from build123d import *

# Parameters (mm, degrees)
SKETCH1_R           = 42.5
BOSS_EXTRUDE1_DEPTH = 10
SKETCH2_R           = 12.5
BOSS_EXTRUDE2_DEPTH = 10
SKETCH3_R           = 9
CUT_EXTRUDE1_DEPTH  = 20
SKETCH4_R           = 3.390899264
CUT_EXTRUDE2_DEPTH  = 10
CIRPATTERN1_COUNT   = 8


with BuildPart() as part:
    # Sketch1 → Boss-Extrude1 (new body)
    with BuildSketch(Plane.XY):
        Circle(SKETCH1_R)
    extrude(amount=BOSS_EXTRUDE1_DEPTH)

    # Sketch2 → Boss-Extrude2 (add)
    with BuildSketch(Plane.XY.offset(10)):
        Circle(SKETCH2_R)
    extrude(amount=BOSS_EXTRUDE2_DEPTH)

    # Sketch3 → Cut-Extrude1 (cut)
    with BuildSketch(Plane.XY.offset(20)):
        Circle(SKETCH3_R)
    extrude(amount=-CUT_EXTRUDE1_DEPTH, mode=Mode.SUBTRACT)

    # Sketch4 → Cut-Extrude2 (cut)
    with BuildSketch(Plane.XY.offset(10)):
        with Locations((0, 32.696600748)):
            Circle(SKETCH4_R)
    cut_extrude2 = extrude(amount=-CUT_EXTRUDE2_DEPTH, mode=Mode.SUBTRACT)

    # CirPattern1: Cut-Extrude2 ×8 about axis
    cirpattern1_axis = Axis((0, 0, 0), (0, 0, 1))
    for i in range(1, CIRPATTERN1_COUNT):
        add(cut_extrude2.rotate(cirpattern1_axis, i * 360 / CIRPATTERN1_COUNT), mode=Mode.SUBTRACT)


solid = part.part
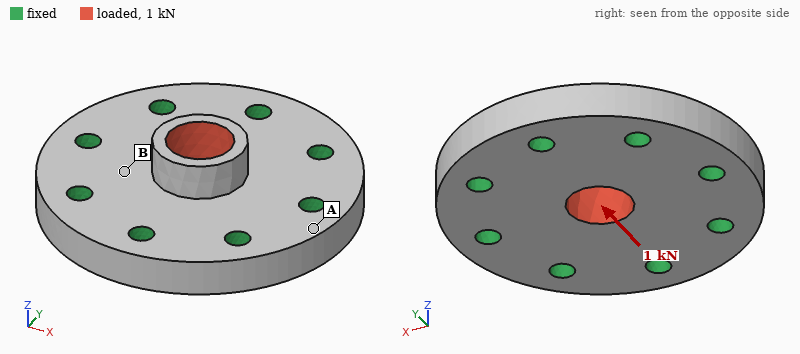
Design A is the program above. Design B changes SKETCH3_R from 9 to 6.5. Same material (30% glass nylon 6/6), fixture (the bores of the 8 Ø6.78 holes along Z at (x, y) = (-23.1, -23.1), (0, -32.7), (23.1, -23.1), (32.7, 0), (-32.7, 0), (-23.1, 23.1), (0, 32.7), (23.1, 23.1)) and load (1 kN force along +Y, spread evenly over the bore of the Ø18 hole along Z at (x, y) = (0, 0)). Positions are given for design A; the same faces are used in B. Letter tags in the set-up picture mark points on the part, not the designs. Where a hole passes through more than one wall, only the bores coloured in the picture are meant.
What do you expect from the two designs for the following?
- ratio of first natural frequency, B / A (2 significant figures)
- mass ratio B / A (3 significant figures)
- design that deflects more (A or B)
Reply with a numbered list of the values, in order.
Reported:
1. 0.94
2. 1.05
3. A
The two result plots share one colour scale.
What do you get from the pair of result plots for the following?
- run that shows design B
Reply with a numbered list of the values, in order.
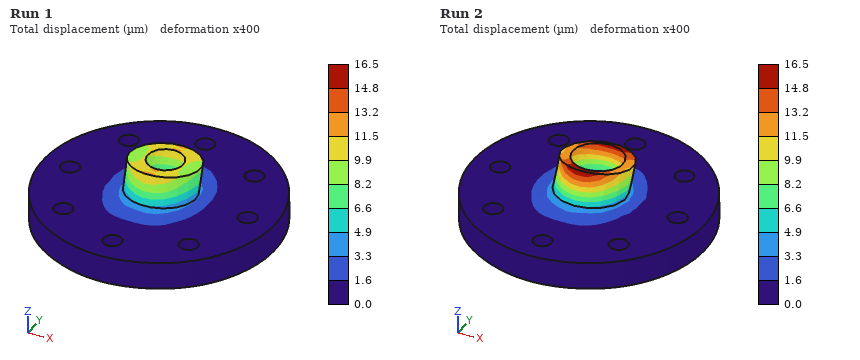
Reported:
1. Run 1
